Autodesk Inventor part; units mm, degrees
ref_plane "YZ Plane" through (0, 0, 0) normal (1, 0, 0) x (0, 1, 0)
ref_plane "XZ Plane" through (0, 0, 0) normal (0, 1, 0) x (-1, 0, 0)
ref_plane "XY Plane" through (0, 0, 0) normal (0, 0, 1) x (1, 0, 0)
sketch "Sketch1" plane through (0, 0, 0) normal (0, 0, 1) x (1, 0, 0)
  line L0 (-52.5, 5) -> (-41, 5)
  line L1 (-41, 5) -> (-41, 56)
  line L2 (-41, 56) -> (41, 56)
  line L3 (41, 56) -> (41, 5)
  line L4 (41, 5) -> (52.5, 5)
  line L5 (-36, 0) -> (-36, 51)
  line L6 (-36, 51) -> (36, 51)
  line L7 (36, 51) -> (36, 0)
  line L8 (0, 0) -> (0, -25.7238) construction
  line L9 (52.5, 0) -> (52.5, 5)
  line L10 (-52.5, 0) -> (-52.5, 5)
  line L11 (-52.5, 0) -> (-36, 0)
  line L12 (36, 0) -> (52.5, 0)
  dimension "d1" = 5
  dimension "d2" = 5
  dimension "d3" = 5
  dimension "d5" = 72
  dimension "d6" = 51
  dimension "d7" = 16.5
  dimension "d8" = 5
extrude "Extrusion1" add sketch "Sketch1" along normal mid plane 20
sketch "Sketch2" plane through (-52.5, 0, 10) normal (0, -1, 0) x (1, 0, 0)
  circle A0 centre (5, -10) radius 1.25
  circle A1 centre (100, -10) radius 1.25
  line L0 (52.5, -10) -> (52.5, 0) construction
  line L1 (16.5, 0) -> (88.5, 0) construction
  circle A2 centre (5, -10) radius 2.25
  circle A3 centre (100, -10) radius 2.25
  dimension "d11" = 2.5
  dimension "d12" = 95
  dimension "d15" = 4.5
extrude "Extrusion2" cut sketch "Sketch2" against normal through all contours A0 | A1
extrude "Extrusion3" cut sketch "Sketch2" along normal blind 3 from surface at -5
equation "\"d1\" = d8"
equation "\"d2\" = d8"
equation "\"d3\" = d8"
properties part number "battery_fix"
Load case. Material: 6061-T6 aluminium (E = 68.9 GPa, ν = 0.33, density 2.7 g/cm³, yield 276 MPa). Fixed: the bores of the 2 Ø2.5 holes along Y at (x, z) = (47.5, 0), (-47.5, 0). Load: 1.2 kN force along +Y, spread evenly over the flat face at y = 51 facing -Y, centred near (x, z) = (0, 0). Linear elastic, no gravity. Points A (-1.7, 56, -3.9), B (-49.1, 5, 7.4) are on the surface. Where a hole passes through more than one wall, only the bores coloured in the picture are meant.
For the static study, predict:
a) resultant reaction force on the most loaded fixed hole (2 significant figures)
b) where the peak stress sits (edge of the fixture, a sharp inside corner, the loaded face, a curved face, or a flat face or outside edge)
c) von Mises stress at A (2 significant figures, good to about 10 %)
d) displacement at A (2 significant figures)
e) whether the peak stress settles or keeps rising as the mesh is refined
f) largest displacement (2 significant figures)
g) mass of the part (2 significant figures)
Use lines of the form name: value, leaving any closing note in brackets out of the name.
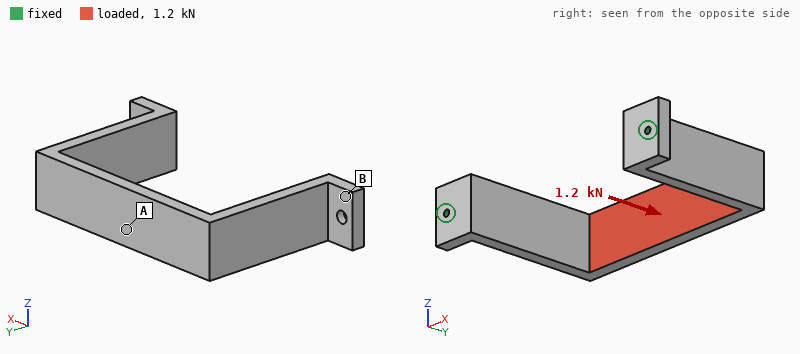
resultant reaction force on the most loaded fixed hole: 640 N
where the peak stress sits: edge of the fixture
von Mises stress at A: 69 MPa
displacement at A: 0.21 mm
whether the peak stress settles or keeps rising as the mesh is refined: keeps rising
largest displacement: 0.21 mm
mass of the part: 56 g
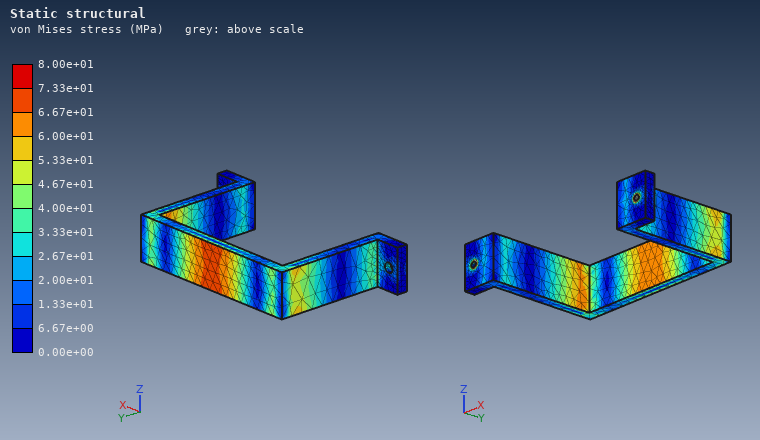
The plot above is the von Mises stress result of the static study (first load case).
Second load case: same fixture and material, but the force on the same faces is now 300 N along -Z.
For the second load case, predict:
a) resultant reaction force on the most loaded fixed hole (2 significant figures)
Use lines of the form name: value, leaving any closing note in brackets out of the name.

resultant reaction force on the most loaded fixed hole: 150 N
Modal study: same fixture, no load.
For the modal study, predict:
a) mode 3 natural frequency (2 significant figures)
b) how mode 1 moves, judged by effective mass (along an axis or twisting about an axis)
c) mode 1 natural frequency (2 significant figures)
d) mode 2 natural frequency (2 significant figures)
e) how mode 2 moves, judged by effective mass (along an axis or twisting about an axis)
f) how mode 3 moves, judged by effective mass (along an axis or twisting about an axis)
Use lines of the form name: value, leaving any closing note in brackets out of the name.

mode 3 natural frequency: 1300 Hz
how mode 1 moves, judged by effective mass: along Z
mode 1 natural frequency: 560 Hz
mode 2 natural frequency: 870 Hz
how mode 2 moves, judged by effective mass: along X
how mode 3 moves, judged by effective mass: twisting about Y
